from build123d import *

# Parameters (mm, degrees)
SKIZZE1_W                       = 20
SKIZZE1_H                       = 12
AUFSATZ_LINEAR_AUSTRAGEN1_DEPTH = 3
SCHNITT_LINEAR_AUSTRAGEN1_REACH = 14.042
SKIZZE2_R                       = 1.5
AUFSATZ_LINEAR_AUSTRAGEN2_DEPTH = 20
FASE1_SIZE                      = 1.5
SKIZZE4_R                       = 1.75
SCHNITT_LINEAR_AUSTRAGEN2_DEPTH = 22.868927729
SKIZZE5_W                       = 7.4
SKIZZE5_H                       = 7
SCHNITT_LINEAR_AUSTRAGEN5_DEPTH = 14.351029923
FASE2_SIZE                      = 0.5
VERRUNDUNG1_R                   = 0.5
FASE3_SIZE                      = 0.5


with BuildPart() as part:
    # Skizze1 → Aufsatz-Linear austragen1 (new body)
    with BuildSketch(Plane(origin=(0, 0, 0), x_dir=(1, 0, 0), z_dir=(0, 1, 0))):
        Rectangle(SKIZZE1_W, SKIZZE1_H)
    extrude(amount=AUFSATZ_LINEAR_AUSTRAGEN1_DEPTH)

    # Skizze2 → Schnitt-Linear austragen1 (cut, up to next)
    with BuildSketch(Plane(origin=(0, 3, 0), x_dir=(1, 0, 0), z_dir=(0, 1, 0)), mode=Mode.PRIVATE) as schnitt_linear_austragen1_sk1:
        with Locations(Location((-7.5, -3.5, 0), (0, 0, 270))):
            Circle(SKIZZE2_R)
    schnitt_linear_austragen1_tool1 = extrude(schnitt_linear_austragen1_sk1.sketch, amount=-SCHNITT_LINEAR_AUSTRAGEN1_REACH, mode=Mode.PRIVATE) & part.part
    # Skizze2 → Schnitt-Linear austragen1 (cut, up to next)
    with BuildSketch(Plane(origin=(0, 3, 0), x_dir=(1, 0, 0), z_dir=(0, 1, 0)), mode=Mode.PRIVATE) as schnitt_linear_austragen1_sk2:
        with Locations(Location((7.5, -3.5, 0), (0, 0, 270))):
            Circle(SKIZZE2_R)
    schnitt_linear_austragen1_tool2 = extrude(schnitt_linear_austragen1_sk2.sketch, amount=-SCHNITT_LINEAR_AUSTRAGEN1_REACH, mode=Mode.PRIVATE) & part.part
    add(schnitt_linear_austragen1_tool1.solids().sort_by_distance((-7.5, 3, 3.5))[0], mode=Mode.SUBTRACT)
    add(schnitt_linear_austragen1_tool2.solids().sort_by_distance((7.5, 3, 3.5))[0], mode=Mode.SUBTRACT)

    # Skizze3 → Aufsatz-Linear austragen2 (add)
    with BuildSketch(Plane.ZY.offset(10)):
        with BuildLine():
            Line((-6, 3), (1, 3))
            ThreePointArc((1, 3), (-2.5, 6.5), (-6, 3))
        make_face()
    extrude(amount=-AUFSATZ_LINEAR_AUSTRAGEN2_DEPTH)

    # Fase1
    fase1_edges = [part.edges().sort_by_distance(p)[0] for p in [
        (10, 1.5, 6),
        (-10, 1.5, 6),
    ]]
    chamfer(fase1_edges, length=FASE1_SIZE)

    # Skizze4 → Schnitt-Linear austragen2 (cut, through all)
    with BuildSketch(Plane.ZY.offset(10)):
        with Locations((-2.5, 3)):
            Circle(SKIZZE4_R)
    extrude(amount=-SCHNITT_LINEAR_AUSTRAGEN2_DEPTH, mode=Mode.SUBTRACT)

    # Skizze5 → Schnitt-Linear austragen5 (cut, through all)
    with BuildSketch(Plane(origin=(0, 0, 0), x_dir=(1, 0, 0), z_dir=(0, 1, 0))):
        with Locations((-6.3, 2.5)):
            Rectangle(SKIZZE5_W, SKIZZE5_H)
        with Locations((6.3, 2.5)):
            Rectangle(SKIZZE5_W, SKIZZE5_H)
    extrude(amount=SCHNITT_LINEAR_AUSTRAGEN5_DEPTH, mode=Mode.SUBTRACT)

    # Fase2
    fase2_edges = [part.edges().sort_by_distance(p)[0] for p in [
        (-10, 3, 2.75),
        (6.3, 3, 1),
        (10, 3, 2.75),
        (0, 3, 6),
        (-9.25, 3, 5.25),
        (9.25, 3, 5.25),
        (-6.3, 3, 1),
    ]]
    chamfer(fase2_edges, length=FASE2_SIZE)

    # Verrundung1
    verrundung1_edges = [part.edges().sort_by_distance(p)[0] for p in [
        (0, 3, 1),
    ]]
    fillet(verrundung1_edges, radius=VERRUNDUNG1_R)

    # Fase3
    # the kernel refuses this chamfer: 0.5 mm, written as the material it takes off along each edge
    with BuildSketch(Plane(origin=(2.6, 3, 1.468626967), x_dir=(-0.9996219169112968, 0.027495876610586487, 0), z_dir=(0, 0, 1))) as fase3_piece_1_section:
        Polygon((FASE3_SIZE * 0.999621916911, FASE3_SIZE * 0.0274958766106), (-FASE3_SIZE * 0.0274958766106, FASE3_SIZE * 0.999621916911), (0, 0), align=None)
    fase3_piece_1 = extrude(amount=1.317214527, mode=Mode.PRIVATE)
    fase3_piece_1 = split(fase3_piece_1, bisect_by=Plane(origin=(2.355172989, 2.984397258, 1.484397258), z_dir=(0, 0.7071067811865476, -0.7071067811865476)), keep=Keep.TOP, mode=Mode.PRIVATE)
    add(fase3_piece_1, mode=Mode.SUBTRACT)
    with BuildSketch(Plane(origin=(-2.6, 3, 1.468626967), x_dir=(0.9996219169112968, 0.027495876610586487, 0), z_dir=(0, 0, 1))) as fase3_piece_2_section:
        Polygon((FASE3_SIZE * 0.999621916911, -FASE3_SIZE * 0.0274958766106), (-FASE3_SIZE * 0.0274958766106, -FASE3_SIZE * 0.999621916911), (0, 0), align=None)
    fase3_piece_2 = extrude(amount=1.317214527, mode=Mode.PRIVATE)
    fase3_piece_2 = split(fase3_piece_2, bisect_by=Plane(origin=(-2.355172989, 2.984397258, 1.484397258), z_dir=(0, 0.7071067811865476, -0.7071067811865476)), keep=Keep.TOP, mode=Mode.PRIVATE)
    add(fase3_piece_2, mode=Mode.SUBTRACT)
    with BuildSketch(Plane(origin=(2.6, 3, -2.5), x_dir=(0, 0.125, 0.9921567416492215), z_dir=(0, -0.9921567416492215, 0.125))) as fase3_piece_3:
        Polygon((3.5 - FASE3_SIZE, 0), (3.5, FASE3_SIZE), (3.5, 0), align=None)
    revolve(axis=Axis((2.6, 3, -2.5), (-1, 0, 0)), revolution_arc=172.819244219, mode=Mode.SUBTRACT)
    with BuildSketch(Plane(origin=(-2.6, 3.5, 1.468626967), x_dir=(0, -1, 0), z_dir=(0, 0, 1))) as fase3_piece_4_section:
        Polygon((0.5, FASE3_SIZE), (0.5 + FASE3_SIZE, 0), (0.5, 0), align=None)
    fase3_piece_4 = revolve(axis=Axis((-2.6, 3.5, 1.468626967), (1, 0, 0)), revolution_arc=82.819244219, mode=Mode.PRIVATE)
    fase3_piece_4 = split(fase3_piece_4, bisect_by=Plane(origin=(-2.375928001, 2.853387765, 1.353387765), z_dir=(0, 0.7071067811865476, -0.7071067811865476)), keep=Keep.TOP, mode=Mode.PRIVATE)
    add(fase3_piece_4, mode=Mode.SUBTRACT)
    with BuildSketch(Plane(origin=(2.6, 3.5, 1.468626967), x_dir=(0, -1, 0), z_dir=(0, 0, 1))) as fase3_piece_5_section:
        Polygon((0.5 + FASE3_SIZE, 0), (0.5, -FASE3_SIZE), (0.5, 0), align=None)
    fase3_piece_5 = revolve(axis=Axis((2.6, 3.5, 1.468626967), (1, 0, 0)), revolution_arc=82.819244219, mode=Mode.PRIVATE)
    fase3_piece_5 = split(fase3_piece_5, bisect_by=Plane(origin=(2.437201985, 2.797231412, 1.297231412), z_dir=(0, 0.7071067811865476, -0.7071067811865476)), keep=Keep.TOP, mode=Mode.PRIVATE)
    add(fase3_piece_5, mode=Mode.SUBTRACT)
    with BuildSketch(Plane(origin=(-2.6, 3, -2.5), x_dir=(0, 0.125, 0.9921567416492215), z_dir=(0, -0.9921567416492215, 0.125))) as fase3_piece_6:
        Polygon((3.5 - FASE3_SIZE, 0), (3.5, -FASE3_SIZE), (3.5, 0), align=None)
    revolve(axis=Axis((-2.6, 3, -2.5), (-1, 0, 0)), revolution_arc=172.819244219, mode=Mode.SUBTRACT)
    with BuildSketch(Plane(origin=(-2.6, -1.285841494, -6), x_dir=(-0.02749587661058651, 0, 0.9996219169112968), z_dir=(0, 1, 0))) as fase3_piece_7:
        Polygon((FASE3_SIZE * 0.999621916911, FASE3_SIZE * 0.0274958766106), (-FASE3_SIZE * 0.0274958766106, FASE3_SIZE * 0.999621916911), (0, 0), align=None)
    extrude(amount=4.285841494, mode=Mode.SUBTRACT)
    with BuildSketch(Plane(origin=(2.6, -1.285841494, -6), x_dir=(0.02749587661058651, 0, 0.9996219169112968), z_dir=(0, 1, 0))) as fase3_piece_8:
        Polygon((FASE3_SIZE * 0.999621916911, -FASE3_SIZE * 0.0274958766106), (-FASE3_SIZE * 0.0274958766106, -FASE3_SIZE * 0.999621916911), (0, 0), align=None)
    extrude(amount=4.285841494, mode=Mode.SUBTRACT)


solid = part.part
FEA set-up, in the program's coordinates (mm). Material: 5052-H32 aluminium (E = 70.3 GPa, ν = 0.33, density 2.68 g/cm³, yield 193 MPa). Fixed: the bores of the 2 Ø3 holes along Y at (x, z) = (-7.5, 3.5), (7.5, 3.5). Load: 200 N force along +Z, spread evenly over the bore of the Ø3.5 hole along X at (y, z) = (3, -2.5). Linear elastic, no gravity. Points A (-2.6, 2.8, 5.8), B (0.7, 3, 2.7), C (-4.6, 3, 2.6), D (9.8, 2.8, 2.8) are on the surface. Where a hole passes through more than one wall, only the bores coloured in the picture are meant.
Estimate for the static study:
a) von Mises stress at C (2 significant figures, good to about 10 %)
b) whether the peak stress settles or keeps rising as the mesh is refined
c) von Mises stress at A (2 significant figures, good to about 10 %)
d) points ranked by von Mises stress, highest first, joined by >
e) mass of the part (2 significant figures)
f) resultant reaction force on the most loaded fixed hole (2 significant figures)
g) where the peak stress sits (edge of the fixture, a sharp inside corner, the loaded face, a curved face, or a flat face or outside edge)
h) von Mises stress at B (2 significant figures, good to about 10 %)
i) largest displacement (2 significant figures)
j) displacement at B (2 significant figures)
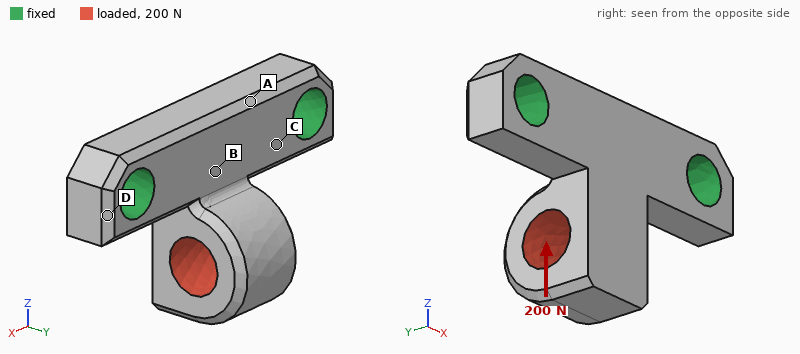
37 MPa
keeps rising
13 MPa
C > B > A > D
1.1 g
100 N
a sharp inside corner
26 MPa
20 µm
4.0 µm
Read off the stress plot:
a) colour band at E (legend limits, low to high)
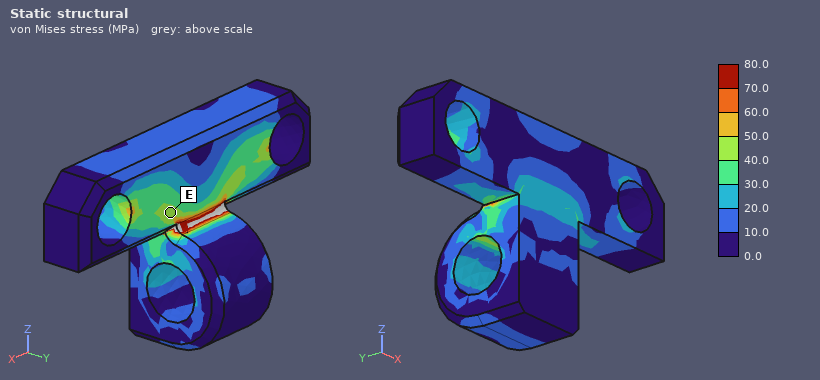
40.0 to 50.0 MPa
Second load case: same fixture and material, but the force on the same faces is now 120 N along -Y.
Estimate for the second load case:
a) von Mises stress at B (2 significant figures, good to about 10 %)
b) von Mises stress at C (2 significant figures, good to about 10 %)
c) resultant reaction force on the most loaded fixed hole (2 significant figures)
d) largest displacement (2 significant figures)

46 MPa
54 MPa
60 N
38 µm
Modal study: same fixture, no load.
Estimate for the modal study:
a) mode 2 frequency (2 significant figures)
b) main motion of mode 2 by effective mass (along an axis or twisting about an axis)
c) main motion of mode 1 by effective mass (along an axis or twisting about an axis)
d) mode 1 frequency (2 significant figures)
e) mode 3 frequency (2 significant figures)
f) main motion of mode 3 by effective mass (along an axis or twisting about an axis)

33 kHz
along X
along Y
15 kHz
51 kHz
along Z
